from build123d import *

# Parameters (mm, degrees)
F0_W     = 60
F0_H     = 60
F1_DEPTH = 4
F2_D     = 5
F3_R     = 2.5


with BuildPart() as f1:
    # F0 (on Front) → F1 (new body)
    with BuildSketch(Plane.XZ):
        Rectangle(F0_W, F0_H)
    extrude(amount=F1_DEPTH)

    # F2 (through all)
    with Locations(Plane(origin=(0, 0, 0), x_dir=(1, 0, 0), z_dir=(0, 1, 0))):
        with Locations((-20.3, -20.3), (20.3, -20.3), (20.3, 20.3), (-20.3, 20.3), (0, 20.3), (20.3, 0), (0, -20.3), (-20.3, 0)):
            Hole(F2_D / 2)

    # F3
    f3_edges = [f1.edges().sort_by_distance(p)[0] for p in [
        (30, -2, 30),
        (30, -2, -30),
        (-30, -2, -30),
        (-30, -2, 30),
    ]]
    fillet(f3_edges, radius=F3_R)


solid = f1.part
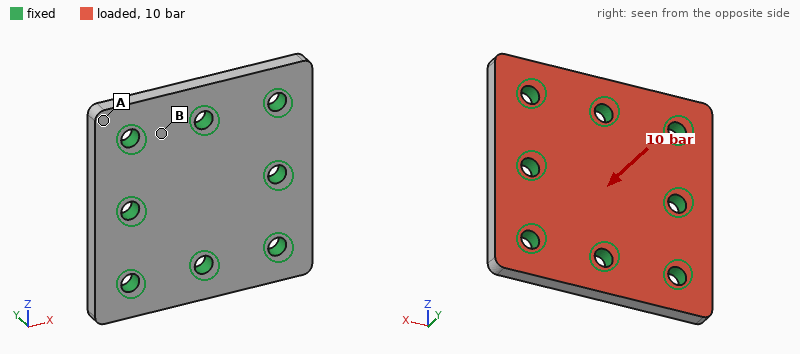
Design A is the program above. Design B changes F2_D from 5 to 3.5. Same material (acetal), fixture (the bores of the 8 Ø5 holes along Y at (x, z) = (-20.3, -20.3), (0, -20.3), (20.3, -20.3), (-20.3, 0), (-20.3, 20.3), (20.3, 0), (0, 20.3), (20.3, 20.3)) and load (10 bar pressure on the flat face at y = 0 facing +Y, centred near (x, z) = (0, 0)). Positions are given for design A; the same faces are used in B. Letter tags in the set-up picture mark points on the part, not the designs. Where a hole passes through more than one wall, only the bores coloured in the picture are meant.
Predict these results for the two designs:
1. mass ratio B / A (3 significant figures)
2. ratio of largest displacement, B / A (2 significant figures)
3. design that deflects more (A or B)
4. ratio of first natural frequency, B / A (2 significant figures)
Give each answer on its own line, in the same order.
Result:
1.02
1.2
B
0.90
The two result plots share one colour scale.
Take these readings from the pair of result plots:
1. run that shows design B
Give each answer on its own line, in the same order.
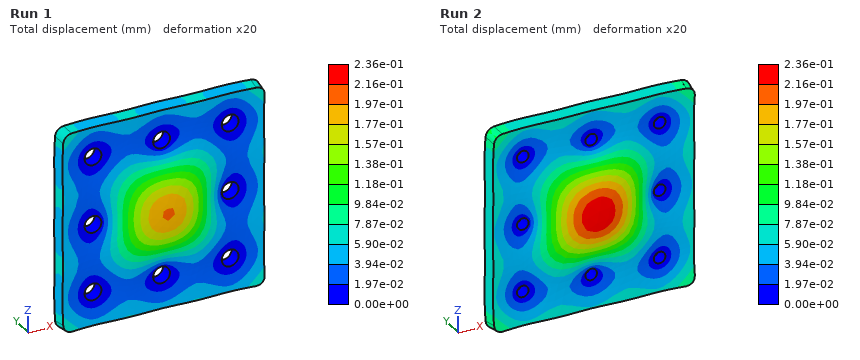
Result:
Run 2
